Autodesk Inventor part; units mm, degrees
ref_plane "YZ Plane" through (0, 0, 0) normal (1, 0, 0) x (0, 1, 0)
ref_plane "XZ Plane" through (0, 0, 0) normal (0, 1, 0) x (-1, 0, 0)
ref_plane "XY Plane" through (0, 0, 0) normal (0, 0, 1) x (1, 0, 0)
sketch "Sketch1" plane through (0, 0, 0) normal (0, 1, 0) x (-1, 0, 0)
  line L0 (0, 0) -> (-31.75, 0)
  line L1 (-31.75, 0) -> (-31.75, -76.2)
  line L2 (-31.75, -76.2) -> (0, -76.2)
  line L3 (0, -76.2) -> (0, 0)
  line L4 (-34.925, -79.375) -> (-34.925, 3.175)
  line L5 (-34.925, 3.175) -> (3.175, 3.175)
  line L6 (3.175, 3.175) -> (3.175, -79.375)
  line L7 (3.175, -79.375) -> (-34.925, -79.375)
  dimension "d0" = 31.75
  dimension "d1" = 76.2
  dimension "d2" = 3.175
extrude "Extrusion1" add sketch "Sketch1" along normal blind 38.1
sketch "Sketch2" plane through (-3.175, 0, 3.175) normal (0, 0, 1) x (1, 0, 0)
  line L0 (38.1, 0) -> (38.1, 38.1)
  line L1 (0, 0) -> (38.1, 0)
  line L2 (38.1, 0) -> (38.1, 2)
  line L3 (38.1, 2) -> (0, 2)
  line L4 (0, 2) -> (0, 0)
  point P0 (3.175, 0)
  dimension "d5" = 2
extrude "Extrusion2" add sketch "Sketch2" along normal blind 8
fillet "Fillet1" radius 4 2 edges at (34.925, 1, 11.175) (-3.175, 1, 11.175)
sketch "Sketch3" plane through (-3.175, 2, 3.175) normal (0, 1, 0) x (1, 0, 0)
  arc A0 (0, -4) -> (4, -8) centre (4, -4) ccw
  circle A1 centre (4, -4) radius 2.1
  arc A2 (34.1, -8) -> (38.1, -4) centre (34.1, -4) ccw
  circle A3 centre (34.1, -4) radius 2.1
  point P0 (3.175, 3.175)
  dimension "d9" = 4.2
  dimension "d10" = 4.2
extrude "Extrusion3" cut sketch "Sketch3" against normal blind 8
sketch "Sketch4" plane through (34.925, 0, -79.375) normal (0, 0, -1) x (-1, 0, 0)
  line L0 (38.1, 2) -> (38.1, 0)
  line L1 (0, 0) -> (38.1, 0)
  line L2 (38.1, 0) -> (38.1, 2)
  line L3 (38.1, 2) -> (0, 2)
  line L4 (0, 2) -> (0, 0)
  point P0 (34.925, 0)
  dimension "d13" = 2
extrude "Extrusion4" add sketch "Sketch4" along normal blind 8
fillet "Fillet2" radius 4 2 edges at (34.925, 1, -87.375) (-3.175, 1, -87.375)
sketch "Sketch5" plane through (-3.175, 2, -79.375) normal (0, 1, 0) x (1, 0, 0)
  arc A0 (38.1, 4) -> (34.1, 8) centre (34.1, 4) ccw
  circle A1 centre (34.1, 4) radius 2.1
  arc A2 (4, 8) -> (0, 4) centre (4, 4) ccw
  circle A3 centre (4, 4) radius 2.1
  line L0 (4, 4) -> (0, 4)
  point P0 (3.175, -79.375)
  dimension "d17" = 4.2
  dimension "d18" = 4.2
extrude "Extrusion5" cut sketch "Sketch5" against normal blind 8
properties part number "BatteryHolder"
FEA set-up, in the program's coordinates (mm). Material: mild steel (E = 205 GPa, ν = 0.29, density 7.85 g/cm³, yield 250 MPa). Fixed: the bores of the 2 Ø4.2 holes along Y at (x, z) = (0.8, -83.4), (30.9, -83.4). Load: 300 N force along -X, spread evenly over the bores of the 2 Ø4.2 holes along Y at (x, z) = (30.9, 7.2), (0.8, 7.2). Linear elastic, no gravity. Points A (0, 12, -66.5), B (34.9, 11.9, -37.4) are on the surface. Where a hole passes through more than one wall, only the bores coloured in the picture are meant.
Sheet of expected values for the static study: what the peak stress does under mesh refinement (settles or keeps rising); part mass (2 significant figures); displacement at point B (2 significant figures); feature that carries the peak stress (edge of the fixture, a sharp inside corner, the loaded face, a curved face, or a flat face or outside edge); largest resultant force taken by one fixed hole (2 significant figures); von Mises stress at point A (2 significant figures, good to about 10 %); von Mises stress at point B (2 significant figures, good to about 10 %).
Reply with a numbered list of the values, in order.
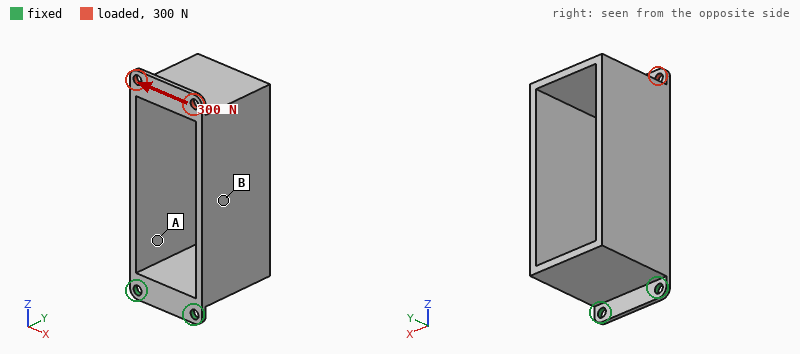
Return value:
1. keeps rising
2. 230 g
3. 0.28 mm
4. a sharp inside corner
5. 800 N
6. 76 MPa
7. 47 MPa
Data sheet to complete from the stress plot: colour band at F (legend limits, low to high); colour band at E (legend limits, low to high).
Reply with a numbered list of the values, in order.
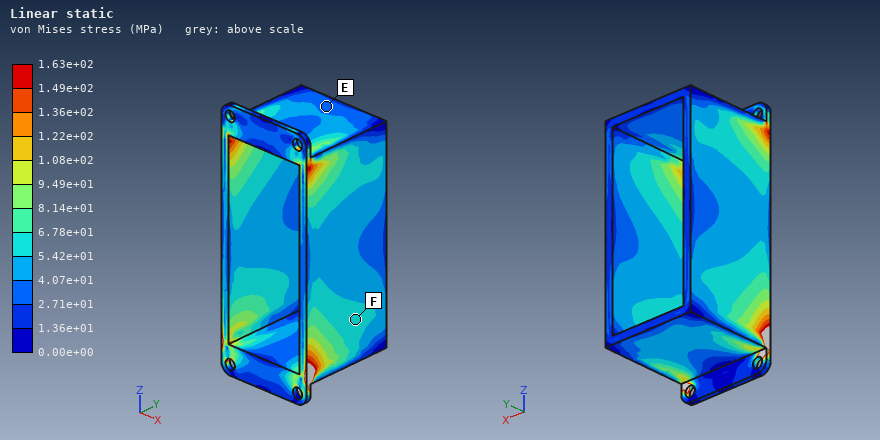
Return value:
1. 5.42e+01 to 6.78e+01 MPa
2. 2.71e+01 to 4.07e+01 MPa
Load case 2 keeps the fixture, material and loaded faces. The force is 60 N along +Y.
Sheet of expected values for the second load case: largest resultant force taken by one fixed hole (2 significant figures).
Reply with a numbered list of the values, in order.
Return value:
1. 64 N
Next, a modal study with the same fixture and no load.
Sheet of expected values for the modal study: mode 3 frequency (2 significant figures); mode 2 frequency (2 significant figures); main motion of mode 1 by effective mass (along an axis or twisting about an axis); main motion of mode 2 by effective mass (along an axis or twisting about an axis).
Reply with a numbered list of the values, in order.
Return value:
1. 1100 Hz
2. 430 Hz
3. along Y
4. along X
